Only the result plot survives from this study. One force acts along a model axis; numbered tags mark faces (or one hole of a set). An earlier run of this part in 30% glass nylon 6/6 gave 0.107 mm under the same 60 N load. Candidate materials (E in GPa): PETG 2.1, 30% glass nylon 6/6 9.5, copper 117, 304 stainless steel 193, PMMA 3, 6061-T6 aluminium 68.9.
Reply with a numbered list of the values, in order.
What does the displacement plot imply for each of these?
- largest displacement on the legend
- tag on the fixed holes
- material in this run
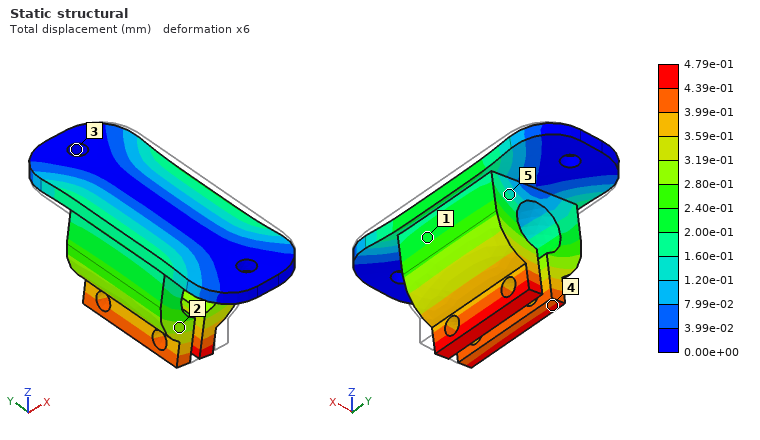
1. 4.79e-01 mm
2. 3
3. PETG
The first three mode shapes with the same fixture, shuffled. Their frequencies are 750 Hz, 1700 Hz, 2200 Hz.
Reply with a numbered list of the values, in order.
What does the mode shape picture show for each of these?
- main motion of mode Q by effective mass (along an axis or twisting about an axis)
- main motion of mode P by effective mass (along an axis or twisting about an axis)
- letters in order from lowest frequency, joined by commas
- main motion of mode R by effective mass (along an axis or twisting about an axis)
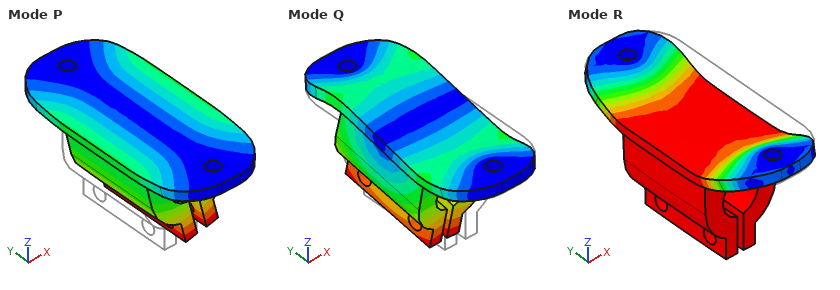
1. along Y
2. along X
3. P, R, Q
4. along Z
